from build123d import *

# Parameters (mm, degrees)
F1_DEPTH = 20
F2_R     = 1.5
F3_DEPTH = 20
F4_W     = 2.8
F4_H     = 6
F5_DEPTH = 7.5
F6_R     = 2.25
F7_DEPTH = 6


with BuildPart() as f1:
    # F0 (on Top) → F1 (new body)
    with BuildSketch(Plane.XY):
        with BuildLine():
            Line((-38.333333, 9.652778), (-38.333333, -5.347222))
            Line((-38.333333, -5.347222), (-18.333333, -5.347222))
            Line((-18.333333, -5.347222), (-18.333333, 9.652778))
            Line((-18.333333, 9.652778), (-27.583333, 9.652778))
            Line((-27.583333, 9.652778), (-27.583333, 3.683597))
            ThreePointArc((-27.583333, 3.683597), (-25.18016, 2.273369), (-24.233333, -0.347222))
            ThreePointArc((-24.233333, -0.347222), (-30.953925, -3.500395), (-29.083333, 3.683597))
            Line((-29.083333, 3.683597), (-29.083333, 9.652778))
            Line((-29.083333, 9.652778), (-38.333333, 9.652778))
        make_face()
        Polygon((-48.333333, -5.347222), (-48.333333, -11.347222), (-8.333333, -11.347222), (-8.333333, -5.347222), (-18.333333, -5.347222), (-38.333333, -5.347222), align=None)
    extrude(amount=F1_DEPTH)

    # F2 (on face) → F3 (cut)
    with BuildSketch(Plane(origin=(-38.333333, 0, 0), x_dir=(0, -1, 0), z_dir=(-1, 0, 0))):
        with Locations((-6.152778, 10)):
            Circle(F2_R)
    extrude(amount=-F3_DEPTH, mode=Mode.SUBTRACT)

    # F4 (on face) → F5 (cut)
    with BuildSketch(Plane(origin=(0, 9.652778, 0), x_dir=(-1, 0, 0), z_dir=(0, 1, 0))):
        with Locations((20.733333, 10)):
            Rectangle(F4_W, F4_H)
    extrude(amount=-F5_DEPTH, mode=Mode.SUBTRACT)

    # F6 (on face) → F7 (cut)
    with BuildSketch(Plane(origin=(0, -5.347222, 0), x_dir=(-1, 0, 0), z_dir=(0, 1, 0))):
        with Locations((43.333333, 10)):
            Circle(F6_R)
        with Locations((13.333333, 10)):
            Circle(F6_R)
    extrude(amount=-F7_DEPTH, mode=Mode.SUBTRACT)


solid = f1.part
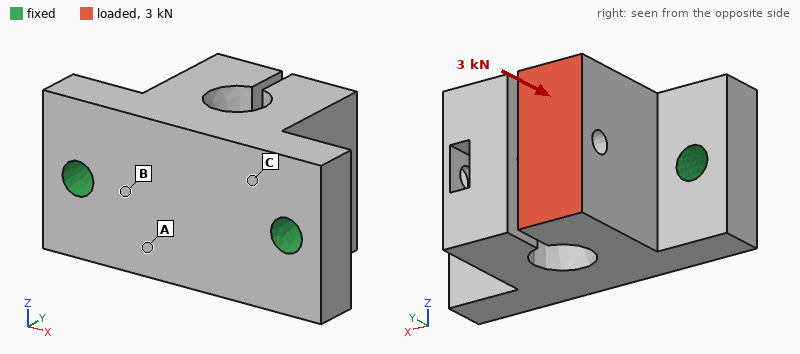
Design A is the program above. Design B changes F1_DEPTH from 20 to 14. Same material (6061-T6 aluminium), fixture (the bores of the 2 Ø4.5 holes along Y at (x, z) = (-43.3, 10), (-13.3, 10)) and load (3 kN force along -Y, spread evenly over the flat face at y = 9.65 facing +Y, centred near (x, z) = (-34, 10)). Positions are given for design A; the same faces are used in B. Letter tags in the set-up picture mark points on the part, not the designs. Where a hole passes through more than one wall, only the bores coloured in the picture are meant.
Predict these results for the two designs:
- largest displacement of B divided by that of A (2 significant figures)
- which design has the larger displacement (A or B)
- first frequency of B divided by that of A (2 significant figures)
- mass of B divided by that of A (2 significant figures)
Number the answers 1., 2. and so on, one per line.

1. 1.6
2. B
3. 0.99
4. 0.69
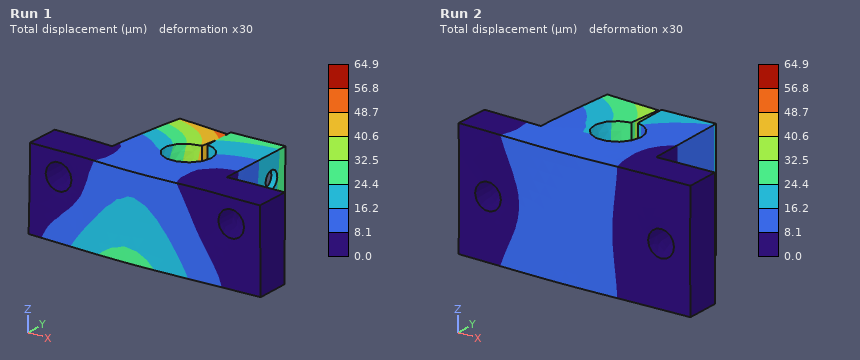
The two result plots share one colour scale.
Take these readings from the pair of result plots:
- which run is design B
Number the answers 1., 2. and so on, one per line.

1. Run 1
